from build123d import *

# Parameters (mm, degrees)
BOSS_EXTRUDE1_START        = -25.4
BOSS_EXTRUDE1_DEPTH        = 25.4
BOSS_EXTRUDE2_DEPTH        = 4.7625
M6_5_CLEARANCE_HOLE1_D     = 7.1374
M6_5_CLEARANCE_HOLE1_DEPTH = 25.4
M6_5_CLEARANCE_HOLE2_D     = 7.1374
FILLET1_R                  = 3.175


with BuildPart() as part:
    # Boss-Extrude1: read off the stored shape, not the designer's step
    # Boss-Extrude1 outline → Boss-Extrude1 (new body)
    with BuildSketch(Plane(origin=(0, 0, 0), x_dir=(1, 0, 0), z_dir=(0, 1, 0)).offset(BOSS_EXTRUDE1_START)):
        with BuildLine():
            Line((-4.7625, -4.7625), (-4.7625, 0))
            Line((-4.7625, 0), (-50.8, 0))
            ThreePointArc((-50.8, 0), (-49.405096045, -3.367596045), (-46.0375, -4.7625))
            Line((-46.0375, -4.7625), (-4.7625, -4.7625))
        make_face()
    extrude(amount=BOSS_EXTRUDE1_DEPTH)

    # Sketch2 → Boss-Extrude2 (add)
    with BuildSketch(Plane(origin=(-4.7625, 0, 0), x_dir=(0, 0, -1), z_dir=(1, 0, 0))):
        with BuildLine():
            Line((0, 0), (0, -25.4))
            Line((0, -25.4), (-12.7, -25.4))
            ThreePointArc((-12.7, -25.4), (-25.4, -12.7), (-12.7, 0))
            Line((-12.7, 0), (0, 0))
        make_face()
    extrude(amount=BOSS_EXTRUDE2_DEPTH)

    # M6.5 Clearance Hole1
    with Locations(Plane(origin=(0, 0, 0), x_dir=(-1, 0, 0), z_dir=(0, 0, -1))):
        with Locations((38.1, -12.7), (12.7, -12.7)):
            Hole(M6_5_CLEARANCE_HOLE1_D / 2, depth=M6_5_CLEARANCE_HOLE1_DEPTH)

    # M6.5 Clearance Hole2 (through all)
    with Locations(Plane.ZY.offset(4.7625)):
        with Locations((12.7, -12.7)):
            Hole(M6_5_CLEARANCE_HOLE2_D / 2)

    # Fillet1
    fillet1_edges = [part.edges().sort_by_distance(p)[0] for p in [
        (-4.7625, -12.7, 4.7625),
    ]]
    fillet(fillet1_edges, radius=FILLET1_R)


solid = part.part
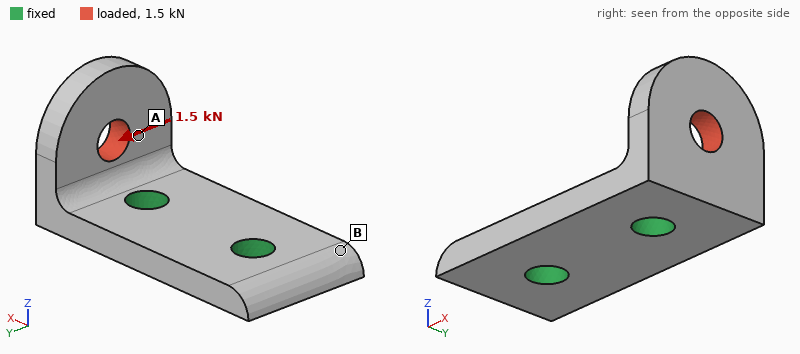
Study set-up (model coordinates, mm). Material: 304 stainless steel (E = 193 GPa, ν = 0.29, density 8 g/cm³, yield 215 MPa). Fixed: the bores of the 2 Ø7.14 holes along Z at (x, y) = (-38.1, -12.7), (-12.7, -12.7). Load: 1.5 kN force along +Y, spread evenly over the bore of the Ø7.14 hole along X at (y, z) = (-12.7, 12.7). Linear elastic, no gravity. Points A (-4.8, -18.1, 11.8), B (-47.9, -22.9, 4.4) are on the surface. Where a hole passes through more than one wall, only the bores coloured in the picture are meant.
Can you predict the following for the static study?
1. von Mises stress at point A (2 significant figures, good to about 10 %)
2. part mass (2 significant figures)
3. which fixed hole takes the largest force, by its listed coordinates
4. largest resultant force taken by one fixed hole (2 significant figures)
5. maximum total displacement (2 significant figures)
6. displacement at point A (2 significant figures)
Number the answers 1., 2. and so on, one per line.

1. 47 MPa
2. 61 g
3. (-12.7, -12.7)
4. 1.8 kN
5. 35 µm
6. 17 µm
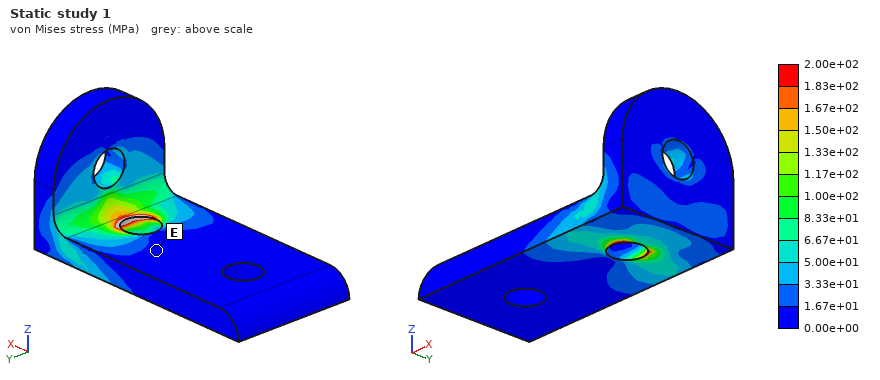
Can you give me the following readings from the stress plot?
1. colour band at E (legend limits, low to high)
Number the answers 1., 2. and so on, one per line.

1. 0.00e+00 to 1.67e+01 MPa
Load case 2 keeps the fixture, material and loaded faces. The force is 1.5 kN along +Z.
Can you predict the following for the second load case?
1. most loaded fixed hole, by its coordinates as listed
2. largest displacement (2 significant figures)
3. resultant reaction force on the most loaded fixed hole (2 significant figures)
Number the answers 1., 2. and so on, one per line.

1. (-12.7, -12.7)
2. 33 µm
3. 1.6 kN
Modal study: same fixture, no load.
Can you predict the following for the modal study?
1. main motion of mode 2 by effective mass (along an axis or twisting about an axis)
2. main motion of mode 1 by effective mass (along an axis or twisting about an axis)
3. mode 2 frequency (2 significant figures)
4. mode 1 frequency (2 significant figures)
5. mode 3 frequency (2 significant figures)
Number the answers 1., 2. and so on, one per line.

1. along Y
2. along X
3. 8300 Hz
4. 5900 Hz
5. 17 kHz
